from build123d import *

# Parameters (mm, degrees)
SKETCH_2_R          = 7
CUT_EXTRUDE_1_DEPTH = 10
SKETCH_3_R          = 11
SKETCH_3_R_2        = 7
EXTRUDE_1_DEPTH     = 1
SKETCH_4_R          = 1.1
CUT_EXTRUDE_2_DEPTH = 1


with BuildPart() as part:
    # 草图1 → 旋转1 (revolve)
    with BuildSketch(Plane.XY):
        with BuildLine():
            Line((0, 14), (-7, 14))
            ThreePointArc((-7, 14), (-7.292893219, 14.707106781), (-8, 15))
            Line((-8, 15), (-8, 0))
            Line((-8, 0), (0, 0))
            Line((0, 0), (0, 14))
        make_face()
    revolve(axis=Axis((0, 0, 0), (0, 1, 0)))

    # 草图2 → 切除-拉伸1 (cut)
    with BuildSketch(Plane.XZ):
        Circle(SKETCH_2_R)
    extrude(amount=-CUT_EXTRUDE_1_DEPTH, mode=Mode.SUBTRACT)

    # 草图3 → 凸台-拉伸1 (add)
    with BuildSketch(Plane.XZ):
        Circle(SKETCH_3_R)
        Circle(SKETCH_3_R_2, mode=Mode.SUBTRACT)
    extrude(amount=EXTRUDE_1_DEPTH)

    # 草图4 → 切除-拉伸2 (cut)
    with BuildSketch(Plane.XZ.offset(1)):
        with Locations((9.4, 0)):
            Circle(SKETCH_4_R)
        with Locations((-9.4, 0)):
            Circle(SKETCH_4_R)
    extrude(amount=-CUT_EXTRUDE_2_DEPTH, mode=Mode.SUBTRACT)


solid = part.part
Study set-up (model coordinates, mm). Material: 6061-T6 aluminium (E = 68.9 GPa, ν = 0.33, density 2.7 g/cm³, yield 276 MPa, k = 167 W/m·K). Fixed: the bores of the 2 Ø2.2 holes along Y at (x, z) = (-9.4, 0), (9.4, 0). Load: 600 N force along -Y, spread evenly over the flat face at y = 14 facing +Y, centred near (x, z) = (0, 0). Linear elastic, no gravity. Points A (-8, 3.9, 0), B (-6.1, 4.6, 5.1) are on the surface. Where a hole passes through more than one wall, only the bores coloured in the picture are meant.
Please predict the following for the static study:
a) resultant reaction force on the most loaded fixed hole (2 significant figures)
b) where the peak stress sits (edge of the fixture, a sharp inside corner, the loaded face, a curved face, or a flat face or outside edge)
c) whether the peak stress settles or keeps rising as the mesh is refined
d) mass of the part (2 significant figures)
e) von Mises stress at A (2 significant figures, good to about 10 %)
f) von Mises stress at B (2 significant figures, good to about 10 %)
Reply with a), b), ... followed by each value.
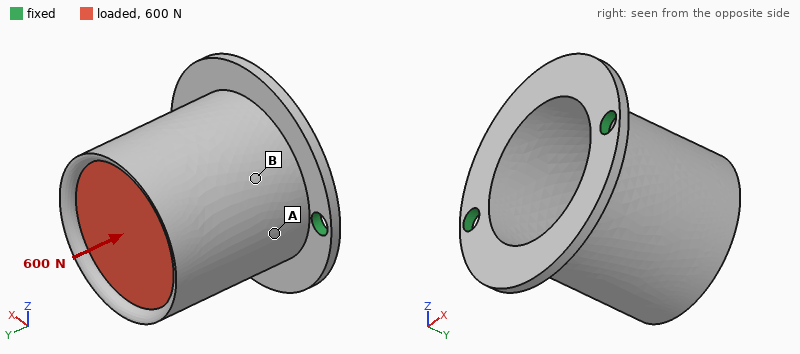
a) 310 N
b) edge of the fixture
c) keeps rising
d) 4.1 g
e) 42 MPa
f) 16 MPa
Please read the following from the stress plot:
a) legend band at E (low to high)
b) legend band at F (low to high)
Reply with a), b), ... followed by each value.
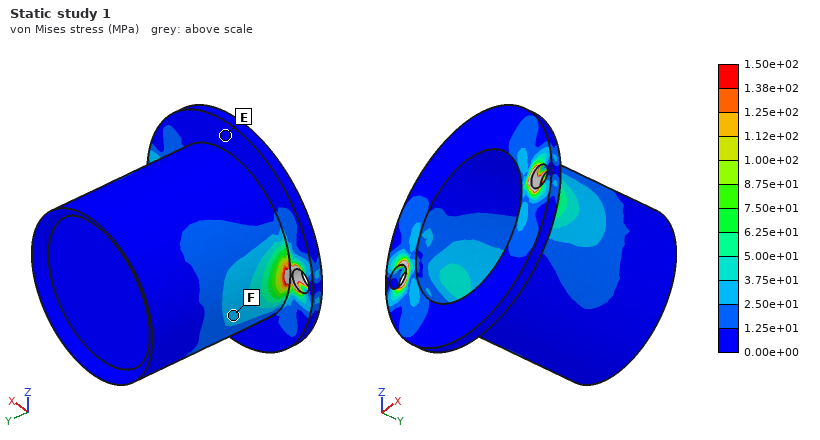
a) 0.00e+00 to 1.25e+01 MPa
b) 2.50e+01 to 3.75e+01 MPa
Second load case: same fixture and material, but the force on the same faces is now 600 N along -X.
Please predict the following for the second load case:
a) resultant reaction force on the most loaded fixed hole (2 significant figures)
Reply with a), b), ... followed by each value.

a) 620 N
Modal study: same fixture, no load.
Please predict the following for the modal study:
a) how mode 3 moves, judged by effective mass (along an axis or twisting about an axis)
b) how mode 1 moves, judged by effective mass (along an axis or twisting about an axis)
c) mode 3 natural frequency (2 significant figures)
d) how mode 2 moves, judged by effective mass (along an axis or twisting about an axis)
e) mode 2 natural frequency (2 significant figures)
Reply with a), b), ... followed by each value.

a) along Y
b) along Z
c) 19 kHz
d) along X
e) 12 kHz
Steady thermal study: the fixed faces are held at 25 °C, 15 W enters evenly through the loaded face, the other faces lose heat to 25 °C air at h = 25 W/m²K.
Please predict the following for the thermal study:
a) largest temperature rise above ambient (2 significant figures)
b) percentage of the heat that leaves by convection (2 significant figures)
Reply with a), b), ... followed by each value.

a) 38 K
b) 7.9 %
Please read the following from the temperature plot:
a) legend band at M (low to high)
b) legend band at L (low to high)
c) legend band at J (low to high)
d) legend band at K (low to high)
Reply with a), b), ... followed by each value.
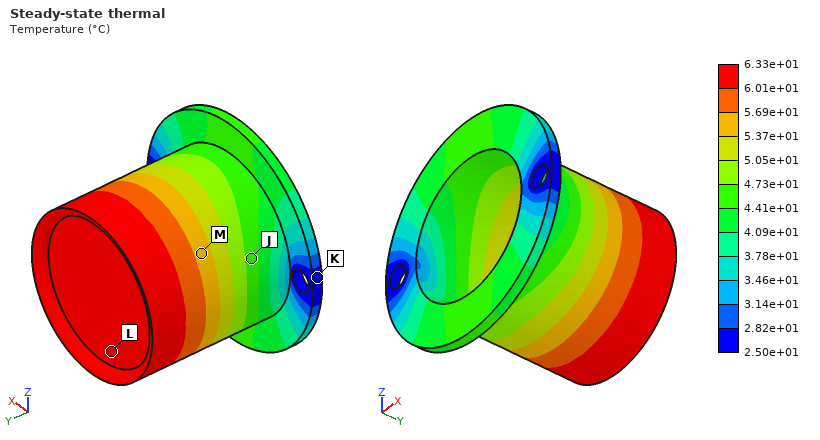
a) 5.37e+01 to 5.69e+01 °C
b) 6.01e+01 to 6.33e+01 °C
c) 4.41e+01 to 4.73e+01 °C
d) 2.50e+01 to 2.82e+01 °C
